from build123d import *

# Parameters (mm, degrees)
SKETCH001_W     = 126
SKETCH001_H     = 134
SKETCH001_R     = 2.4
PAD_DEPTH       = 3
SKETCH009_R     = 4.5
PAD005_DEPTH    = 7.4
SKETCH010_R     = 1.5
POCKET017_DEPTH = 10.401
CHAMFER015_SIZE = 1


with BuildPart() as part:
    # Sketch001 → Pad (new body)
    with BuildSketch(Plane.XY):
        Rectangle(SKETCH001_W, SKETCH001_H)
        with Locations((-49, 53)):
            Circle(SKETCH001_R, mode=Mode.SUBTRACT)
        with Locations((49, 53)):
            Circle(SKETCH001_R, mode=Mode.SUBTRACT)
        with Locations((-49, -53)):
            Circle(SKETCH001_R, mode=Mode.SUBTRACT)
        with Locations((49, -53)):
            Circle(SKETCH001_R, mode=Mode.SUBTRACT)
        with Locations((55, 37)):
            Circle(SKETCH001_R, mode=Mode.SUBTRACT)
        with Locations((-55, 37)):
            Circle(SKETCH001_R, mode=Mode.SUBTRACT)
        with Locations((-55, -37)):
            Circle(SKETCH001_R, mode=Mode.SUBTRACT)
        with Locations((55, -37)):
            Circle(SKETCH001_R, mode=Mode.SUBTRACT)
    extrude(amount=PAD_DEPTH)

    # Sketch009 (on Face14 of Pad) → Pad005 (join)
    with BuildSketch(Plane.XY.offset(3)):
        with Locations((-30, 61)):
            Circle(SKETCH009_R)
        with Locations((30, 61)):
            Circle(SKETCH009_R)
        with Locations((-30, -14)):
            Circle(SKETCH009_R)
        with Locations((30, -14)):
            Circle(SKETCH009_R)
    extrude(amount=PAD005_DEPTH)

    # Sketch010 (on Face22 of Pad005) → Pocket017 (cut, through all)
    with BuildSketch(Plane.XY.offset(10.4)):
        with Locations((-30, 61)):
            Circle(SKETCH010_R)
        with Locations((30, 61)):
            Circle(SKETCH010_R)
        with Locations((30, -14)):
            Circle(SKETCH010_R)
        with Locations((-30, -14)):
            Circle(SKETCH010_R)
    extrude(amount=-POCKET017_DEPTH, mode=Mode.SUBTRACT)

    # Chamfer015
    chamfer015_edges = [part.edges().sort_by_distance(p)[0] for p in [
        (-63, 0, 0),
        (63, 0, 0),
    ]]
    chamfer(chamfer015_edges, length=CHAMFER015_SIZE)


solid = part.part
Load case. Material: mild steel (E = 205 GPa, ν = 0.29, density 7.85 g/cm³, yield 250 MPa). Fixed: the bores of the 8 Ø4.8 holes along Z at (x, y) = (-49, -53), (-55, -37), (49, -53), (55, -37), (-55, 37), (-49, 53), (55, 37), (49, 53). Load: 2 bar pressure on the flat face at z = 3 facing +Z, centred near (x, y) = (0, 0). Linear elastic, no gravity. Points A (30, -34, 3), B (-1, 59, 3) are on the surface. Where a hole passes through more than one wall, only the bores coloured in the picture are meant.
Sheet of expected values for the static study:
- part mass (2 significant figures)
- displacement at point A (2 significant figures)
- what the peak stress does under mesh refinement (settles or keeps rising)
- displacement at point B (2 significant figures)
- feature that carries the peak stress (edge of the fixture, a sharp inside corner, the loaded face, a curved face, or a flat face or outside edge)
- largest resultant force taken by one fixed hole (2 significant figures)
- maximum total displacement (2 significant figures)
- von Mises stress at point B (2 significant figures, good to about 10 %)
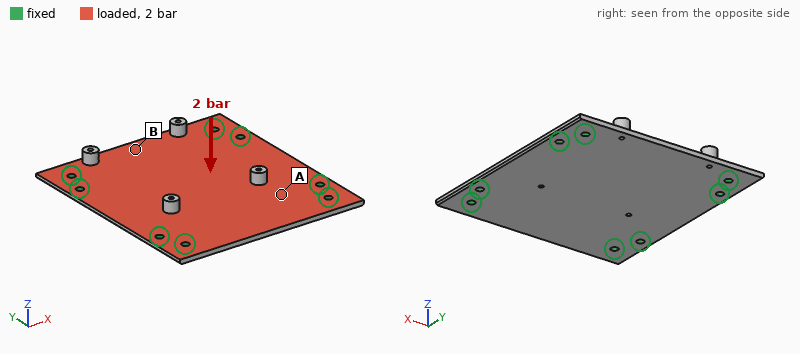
410 g
0.083 mm
keeps rising
0.12 mm
edge of the fixture
460 N
0.21 mm
63 MPa
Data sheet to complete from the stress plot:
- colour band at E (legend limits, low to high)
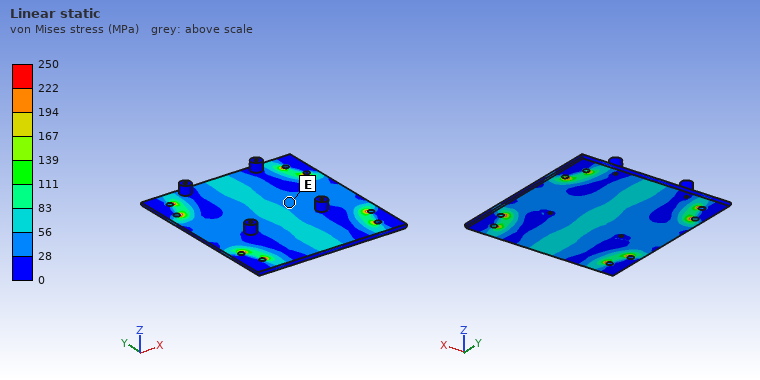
28 to 56 MPa
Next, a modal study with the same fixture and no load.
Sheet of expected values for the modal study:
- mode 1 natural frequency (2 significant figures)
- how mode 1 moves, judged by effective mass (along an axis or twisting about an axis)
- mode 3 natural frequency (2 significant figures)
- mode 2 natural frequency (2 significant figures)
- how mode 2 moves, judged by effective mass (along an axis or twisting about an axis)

1200 Hz
along Z
2100 Hz
1800 Hz
twisting about X
